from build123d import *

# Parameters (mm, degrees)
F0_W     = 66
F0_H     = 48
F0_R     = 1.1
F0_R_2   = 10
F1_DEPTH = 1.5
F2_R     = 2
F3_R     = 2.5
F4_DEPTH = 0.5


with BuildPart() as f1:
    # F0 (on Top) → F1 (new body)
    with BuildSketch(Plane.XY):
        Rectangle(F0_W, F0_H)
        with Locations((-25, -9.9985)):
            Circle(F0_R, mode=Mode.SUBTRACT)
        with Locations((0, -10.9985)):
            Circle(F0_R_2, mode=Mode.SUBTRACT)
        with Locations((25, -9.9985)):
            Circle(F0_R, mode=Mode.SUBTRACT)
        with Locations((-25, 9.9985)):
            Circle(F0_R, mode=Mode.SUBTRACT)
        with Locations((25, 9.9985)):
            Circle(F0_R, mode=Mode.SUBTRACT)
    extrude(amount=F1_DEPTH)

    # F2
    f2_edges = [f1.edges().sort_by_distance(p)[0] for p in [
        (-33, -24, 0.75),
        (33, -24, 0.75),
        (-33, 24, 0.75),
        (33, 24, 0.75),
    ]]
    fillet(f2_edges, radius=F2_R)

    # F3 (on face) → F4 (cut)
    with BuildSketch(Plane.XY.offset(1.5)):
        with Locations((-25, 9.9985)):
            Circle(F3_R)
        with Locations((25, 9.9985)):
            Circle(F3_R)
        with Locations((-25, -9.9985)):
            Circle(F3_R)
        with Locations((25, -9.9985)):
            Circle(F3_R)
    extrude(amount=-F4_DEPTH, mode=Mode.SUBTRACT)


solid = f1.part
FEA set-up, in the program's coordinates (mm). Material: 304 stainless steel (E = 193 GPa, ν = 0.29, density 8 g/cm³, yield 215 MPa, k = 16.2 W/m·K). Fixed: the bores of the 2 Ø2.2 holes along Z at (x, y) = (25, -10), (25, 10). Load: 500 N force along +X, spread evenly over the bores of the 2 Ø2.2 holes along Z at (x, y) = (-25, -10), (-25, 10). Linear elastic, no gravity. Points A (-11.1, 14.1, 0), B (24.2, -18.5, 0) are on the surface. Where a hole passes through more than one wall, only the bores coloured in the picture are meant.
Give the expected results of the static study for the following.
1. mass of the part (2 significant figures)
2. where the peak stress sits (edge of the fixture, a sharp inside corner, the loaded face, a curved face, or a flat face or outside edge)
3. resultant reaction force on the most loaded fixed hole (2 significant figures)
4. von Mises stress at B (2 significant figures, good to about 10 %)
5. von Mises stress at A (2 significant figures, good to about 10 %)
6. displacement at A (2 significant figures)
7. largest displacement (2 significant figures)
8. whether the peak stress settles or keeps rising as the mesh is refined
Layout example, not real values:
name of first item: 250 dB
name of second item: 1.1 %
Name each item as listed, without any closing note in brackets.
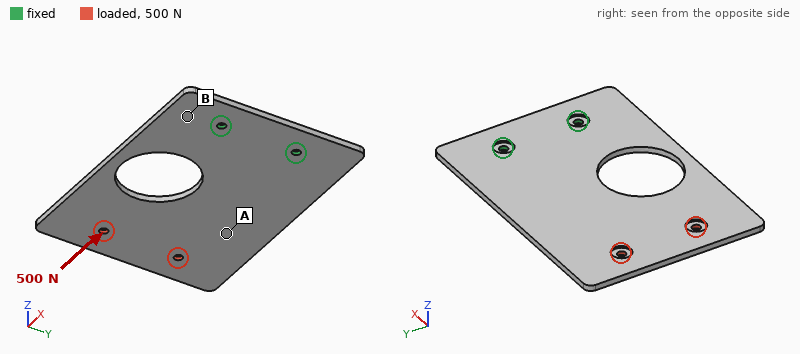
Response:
mass of the part: 34 g
where the peak stress sits: edge of the fixture
resultant reaction force on the most loaded fixed hole: 250 N
von Mises stress at B: 8.2 MPa
von Mises stress at A: 17 MPa
displacement at A: 37 µm
largest displacement: 100 µm
whether the peak stress settles or keeps rising as the mesh is refined: keeps rising
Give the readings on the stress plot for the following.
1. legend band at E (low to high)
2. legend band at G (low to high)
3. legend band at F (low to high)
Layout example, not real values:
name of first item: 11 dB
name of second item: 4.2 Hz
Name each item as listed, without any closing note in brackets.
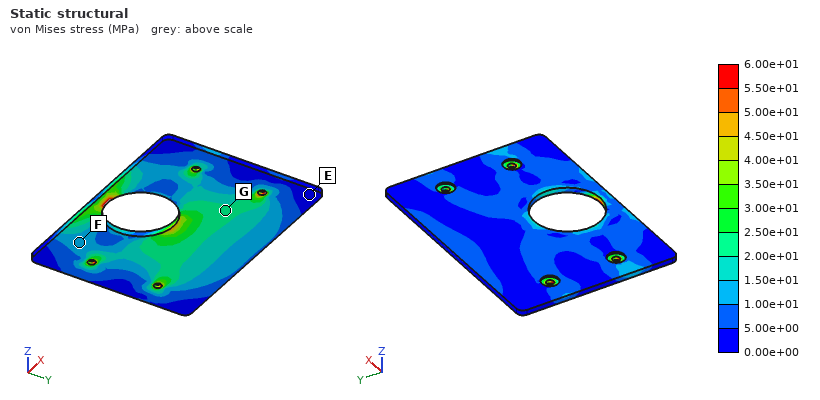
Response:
legend band at E: 0.00e+00 to 5.00e+00 MPa
legend band at G: 2.00e+01 to 2.50e+01 MPa
legend band at F: 1.00e+01 to 1.50e+01 MPa
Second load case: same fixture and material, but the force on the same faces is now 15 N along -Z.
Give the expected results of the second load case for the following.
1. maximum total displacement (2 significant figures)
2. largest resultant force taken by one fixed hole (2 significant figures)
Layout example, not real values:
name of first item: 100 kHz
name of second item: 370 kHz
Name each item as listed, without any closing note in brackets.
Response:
maximum total displacement: 0.46 mm
largest resultant force taken by one fixed hole: 13 N
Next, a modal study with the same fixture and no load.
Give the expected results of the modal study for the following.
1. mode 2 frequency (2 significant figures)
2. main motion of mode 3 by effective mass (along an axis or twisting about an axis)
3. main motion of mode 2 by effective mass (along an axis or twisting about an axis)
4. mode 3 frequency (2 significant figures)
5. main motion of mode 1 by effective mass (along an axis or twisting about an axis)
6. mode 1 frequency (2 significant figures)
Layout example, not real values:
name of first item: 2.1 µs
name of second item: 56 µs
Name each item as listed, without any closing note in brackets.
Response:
mode 2 frequency: 850 Hz
main motion of mode 3 by effective mass: along Z
main motion of mode 2 by effective mass: twisting about X
mode 3 frequency: 1900 Hz
main motion of mode 1 by effective mass: along Z
mode 1 frequency: 290 Hz
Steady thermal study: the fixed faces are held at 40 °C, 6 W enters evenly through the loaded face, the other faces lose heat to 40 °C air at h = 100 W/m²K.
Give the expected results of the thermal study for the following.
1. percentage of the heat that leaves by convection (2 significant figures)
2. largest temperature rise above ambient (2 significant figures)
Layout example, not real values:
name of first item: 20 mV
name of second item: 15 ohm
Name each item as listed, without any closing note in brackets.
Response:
percentage of the heat that leaves by convection: 100 %
largest temperature rise above ambient: 70 K
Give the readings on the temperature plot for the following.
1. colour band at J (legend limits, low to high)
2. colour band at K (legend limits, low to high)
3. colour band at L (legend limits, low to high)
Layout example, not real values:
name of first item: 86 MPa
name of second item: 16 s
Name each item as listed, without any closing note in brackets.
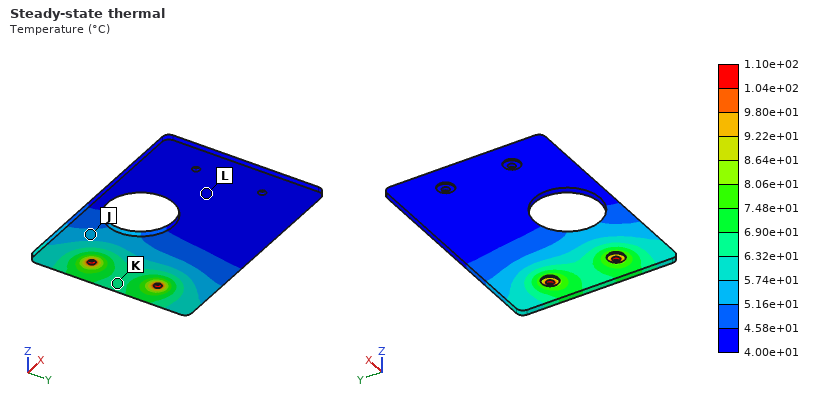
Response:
colour band at J: 5.16e+01 to 5.74e+01 °C
colour band at K: 6.32e+01 to 6.90e+01 °C
colour band at L: 4.00e+01 to 4.58e+01 °C
